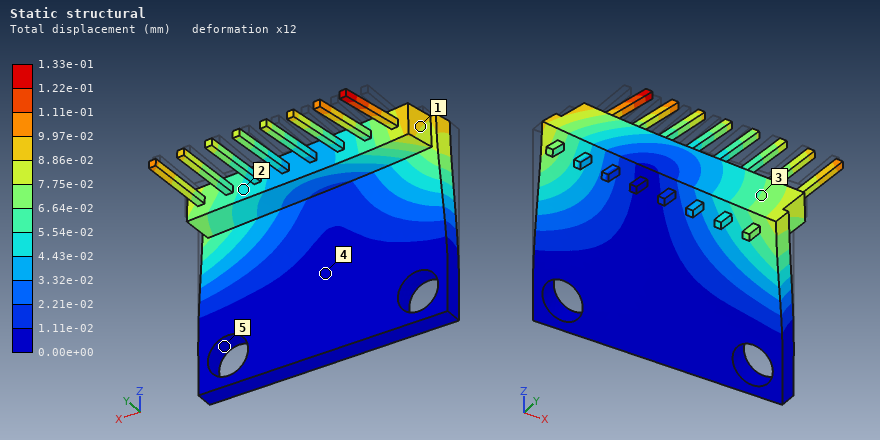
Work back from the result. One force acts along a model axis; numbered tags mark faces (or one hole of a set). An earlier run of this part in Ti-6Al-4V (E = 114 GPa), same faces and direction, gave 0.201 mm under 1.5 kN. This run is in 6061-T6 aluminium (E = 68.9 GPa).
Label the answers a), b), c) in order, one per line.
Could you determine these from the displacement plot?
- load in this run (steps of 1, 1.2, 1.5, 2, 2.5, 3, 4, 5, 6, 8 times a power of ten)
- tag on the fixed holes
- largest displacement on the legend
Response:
a) 600 N
b) 5
c) 1.33e-01 mm
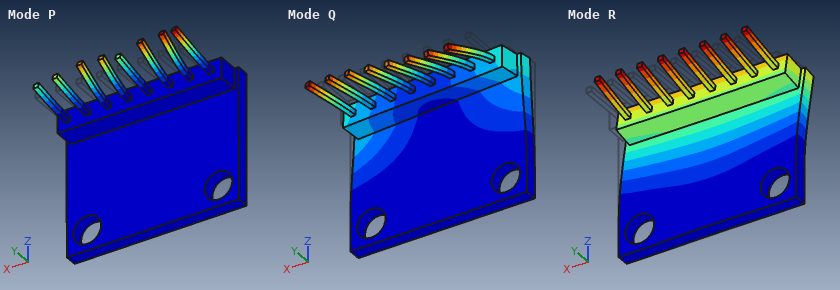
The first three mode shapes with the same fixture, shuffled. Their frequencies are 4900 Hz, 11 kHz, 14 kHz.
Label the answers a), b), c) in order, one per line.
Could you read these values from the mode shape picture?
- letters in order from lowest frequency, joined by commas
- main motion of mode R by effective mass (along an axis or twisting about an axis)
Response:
a) R, Q, P
b) along Y
